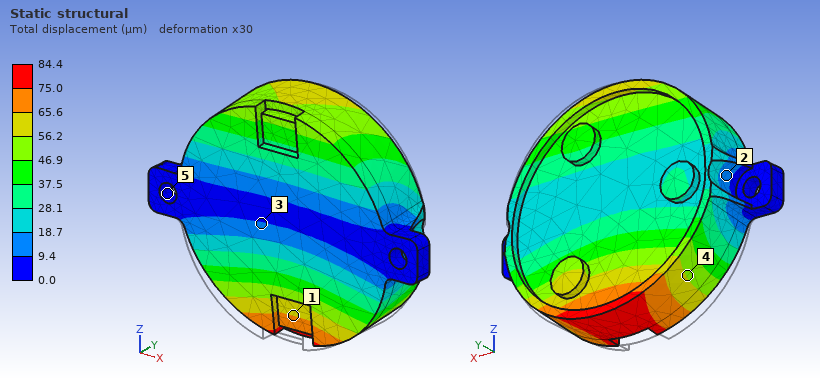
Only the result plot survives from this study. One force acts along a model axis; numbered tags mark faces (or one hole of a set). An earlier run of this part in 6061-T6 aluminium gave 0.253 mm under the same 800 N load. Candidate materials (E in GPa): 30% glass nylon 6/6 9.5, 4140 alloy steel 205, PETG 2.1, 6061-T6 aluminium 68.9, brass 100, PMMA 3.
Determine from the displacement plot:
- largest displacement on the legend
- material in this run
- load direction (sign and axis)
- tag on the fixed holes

84.4 µm
4140 alloy steel
+Y
5
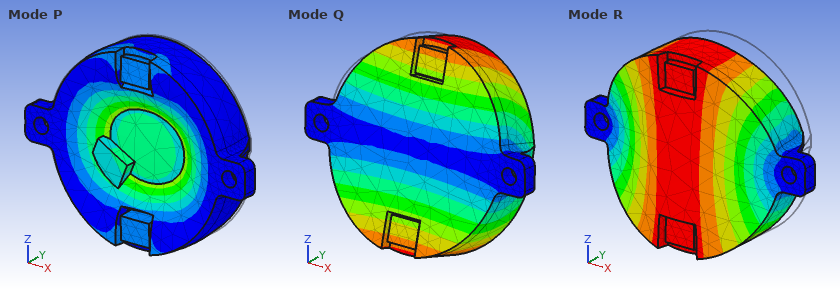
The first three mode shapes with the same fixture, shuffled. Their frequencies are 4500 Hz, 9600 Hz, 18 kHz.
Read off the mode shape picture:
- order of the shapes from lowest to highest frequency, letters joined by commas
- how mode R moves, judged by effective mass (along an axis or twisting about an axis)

Q, R, P
along Y
